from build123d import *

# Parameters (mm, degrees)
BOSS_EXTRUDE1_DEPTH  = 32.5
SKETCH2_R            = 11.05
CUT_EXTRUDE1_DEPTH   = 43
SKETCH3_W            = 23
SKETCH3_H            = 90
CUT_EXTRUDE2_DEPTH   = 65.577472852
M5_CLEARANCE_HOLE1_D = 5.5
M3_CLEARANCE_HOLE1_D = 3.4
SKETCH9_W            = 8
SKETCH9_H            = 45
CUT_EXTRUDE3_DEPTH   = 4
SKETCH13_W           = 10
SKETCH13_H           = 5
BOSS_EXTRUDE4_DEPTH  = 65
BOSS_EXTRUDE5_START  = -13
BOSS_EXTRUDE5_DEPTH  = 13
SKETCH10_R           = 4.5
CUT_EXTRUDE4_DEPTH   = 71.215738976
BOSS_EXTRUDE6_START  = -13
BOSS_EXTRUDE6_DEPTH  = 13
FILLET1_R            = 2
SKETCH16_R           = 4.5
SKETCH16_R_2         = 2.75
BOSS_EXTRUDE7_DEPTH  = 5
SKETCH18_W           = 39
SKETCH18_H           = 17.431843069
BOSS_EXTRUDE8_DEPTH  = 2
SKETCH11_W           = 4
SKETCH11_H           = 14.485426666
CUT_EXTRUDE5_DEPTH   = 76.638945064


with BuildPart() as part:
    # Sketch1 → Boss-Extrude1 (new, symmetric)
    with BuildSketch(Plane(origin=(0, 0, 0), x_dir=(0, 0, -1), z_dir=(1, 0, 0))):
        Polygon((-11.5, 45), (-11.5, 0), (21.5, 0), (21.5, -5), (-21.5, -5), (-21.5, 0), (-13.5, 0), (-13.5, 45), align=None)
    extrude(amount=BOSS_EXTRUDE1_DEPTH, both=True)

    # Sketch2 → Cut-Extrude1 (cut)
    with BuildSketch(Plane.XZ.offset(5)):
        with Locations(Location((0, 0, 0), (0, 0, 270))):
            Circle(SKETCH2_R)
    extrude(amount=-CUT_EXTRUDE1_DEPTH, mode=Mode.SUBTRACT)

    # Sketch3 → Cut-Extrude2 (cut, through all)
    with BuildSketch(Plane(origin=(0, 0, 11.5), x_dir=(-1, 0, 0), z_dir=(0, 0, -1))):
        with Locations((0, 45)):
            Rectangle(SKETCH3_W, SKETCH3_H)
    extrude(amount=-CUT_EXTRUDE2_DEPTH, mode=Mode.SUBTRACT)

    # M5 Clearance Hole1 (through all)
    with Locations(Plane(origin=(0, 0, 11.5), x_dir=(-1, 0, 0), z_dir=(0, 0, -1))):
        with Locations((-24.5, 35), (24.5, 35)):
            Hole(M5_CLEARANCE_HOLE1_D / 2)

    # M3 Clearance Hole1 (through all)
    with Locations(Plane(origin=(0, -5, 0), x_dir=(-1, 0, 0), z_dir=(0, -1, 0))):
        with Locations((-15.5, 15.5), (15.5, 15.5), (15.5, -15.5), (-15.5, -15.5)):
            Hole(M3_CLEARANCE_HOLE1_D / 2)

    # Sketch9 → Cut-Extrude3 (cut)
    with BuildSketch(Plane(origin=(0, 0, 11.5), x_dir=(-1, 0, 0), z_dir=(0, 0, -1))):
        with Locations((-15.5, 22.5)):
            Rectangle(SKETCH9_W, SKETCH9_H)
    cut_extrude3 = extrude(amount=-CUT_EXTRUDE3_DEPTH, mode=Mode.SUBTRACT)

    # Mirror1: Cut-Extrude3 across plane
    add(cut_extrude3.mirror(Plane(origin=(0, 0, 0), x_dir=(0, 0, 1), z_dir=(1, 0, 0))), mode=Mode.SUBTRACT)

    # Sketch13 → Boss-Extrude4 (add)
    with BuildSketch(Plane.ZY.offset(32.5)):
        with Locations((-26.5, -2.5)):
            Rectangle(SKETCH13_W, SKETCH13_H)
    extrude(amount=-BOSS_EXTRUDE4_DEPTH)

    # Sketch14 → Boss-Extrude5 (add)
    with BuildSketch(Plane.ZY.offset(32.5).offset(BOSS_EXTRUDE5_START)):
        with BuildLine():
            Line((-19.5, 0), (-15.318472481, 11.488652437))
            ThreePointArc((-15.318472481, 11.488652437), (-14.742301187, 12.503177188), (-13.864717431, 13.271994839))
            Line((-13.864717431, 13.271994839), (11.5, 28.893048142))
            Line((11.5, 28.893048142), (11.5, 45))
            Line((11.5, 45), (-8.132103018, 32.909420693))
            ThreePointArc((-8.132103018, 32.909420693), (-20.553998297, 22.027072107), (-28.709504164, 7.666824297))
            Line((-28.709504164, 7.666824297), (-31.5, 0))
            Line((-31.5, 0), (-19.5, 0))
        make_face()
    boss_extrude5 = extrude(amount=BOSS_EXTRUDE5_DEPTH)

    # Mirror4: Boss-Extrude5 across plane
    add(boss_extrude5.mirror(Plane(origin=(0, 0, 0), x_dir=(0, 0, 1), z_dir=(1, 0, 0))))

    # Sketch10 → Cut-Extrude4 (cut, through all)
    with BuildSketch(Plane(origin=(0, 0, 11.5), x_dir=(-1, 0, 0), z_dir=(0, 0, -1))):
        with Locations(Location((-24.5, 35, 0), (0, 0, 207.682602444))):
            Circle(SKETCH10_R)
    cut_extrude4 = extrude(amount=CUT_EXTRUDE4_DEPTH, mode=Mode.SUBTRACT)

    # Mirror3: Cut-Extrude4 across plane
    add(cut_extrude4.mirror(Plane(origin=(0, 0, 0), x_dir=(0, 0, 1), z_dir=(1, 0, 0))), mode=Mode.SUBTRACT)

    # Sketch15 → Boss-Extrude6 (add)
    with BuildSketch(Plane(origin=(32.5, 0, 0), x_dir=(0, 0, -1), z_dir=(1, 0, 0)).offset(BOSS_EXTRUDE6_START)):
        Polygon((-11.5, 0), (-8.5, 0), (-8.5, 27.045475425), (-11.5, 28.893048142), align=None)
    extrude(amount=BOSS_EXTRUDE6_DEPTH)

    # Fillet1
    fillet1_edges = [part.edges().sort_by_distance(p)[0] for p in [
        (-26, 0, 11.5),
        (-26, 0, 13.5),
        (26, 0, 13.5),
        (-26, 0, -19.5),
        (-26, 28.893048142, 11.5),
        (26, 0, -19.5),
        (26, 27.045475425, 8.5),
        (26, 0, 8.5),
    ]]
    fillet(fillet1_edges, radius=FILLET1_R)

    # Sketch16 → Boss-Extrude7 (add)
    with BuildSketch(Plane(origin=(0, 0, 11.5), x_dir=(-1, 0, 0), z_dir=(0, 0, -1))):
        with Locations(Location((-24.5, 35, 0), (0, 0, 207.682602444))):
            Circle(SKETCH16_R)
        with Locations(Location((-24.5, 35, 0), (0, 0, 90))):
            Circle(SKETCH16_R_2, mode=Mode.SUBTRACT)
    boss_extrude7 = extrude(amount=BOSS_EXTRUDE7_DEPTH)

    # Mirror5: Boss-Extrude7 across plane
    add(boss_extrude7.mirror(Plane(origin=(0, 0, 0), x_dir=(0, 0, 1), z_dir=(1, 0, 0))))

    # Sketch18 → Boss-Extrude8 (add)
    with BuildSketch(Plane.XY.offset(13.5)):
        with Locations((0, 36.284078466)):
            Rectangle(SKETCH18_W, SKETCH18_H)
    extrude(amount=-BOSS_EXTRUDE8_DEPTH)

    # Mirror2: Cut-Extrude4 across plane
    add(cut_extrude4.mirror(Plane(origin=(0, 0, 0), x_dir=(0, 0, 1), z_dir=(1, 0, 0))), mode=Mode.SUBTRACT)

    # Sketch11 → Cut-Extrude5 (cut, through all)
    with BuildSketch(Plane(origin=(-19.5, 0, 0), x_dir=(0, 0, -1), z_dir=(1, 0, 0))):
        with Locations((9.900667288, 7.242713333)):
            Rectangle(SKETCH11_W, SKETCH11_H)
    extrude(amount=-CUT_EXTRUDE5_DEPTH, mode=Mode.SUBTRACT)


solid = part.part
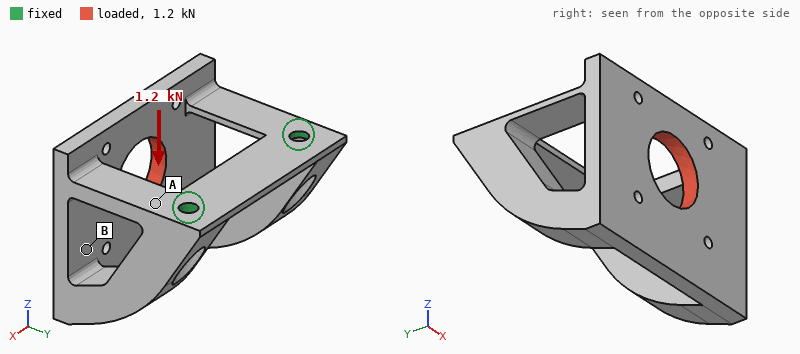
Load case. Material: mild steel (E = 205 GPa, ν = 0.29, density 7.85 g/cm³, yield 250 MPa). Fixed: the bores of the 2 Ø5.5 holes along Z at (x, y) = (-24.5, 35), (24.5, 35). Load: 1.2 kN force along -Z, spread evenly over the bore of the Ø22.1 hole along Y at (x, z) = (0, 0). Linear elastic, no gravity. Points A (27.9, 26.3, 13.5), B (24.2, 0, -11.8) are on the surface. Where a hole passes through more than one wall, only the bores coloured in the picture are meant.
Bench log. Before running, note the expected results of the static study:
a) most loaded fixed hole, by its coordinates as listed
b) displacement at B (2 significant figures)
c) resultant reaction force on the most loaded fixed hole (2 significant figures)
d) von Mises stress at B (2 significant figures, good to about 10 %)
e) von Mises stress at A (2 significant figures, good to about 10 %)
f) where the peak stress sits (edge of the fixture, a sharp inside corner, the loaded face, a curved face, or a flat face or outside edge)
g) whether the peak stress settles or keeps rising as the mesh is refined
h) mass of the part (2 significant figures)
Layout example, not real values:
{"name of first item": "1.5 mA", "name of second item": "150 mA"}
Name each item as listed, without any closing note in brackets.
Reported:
{"most loaded fixed hole, by its coordinates as listed": "(24.5, 35)", "displacement at B": "0.071 mm", "resultant reaction force on the most loaded fixed hole": "780 N", "von Mises stress at B": "24 MPa", "von Mises stress at A": "69 MPa", "where the peak stress sits": "edge of the fixture", "whether the peak stress settles or keeps rising as the mesh is refined": "keeps rising", "mass of the part": "280 g"}
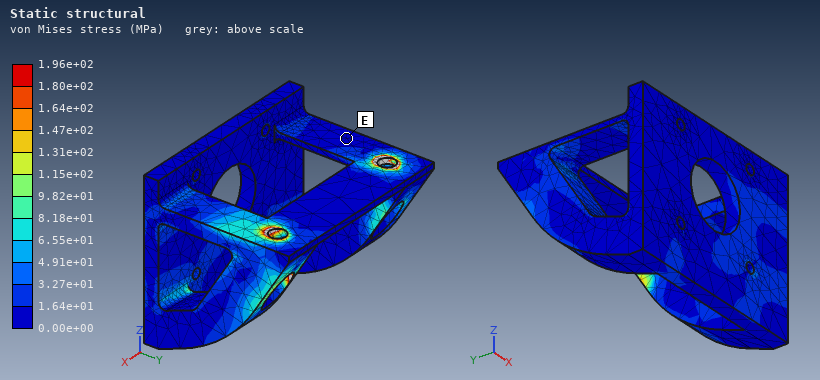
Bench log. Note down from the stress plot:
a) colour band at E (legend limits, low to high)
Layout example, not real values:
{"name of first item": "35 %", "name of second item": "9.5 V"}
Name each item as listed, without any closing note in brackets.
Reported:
{"colour band at E": "0.00e+00 to 1.64e+01 MPa"}
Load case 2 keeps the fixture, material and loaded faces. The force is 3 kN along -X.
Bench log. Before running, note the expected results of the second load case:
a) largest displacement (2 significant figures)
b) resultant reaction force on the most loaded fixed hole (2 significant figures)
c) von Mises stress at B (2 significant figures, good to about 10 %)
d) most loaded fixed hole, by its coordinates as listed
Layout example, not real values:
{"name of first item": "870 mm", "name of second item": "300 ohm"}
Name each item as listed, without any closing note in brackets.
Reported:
{"largest displacement": "85 µm", "resultant reaction force on the most loaded fixed hole": "2.3 kN", "von Mises stress at B": "34 MPa", "most loaded fixed hole, by its coordinates as listed": "(24.5, 35)"}
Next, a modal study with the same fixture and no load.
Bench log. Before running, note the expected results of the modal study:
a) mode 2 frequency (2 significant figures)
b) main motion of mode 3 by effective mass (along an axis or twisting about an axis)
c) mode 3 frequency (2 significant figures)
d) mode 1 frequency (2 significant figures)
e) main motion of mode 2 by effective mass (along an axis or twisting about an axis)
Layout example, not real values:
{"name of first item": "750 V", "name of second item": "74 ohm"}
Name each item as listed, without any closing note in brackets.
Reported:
{"mode 2 frequency": "2100 Hz", "main motion of mode 3 by effective mass": "along X", "mode 3 frequency": "2900 Hz", "mode 1 frequency": "1300 Hz", "main motion of mode 2 by effective mass": "along X"}
